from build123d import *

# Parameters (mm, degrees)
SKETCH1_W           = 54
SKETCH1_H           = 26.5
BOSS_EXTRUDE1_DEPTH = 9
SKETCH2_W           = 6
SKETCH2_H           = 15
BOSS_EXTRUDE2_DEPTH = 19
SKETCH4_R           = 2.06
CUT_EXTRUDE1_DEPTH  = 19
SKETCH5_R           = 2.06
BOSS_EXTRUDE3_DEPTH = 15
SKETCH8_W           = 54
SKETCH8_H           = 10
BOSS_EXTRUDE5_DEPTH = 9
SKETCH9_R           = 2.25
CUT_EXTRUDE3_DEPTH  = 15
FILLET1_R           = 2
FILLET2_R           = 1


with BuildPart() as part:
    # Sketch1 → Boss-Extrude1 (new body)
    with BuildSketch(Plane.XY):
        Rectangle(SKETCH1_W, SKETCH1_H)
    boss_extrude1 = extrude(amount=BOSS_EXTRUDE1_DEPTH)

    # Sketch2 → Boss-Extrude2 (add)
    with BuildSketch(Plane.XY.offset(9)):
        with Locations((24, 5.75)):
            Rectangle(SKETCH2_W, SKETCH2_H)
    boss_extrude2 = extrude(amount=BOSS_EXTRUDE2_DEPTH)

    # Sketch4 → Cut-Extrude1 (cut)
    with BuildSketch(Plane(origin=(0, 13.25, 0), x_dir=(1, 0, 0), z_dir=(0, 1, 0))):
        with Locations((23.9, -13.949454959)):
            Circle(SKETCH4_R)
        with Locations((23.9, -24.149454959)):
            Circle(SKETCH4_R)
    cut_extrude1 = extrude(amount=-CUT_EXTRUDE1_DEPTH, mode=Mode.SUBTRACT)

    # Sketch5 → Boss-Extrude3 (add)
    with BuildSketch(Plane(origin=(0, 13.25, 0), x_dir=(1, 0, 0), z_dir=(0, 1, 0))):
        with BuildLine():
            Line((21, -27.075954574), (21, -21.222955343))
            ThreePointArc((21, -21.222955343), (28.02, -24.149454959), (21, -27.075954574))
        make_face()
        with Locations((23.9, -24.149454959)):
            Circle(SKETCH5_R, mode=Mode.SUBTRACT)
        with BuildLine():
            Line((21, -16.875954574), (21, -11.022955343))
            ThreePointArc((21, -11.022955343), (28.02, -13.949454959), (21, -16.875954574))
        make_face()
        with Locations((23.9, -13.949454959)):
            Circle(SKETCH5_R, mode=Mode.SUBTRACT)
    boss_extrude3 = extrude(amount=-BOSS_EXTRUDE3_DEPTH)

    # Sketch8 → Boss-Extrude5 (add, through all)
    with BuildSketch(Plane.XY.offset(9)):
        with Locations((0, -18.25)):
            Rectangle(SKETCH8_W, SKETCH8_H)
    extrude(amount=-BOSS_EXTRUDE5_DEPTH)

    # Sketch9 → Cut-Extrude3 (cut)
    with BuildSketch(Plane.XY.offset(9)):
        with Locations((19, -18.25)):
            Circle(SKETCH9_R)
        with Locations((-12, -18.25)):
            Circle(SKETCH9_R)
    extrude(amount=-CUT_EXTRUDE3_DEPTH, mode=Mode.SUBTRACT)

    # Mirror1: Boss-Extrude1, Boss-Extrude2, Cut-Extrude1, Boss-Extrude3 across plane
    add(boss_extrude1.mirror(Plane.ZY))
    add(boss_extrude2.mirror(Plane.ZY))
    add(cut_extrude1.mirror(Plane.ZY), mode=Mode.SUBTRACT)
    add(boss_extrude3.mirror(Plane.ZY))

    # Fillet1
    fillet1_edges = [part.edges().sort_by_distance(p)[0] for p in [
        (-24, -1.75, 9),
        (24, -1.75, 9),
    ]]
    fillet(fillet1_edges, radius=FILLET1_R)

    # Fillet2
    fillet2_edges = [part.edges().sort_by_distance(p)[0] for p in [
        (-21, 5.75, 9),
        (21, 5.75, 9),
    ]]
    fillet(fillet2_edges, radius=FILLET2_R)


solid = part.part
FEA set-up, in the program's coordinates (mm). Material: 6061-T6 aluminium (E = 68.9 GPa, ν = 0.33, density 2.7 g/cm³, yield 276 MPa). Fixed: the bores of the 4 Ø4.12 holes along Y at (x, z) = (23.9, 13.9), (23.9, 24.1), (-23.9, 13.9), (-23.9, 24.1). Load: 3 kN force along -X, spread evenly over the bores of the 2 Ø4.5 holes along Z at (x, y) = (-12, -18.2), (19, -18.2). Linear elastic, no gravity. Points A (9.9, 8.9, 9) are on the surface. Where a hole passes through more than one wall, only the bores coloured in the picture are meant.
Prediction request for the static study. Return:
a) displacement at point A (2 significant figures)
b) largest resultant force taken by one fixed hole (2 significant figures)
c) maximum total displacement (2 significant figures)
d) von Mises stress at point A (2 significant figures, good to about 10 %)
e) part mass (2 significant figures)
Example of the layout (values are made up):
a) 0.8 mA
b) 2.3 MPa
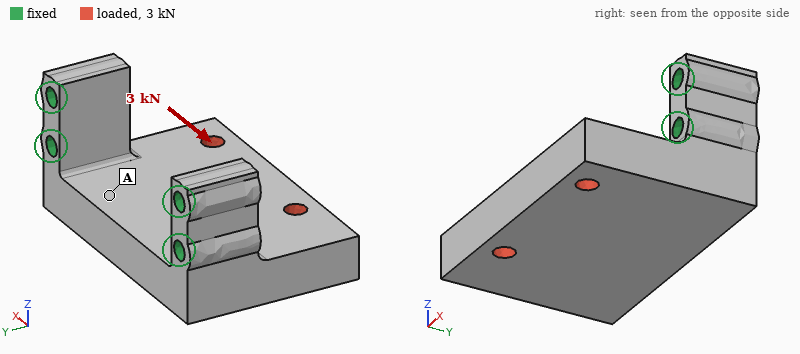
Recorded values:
a) 7.1 µm
b) 2.1 kN
c) 26 µm
d) 12 MPa
e) 55 g
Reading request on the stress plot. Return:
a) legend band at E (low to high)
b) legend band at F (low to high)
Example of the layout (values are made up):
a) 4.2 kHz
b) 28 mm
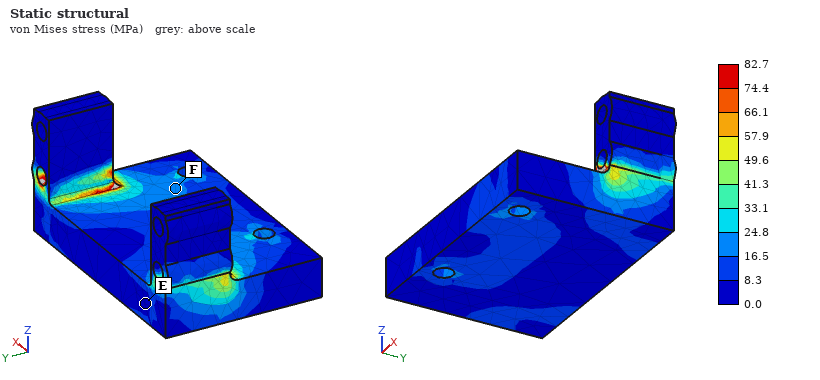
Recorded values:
a) 0.0 to 8.3 MPa
b) 16.5 to 24.8 MPa
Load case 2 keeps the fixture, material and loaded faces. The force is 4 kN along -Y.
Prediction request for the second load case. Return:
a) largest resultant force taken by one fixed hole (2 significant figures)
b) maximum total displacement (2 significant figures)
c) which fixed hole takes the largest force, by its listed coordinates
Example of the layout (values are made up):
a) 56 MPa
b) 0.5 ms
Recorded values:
a) 2.3 kN
b) 32 µm
c) (23.9, 13.9)
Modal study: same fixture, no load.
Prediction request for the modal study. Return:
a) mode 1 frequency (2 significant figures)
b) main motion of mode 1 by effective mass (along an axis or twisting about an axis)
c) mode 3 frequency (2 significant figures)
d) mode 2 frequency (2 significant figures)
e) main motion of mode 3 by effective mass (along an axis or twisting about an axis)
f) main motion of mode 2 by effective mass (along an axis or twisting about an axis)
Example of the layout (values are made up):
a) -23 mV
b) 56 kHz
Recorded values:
a) 5900 Hz
b) along Z
c) 14 kHz
d) 11 kHz
e) along X
f) along X
